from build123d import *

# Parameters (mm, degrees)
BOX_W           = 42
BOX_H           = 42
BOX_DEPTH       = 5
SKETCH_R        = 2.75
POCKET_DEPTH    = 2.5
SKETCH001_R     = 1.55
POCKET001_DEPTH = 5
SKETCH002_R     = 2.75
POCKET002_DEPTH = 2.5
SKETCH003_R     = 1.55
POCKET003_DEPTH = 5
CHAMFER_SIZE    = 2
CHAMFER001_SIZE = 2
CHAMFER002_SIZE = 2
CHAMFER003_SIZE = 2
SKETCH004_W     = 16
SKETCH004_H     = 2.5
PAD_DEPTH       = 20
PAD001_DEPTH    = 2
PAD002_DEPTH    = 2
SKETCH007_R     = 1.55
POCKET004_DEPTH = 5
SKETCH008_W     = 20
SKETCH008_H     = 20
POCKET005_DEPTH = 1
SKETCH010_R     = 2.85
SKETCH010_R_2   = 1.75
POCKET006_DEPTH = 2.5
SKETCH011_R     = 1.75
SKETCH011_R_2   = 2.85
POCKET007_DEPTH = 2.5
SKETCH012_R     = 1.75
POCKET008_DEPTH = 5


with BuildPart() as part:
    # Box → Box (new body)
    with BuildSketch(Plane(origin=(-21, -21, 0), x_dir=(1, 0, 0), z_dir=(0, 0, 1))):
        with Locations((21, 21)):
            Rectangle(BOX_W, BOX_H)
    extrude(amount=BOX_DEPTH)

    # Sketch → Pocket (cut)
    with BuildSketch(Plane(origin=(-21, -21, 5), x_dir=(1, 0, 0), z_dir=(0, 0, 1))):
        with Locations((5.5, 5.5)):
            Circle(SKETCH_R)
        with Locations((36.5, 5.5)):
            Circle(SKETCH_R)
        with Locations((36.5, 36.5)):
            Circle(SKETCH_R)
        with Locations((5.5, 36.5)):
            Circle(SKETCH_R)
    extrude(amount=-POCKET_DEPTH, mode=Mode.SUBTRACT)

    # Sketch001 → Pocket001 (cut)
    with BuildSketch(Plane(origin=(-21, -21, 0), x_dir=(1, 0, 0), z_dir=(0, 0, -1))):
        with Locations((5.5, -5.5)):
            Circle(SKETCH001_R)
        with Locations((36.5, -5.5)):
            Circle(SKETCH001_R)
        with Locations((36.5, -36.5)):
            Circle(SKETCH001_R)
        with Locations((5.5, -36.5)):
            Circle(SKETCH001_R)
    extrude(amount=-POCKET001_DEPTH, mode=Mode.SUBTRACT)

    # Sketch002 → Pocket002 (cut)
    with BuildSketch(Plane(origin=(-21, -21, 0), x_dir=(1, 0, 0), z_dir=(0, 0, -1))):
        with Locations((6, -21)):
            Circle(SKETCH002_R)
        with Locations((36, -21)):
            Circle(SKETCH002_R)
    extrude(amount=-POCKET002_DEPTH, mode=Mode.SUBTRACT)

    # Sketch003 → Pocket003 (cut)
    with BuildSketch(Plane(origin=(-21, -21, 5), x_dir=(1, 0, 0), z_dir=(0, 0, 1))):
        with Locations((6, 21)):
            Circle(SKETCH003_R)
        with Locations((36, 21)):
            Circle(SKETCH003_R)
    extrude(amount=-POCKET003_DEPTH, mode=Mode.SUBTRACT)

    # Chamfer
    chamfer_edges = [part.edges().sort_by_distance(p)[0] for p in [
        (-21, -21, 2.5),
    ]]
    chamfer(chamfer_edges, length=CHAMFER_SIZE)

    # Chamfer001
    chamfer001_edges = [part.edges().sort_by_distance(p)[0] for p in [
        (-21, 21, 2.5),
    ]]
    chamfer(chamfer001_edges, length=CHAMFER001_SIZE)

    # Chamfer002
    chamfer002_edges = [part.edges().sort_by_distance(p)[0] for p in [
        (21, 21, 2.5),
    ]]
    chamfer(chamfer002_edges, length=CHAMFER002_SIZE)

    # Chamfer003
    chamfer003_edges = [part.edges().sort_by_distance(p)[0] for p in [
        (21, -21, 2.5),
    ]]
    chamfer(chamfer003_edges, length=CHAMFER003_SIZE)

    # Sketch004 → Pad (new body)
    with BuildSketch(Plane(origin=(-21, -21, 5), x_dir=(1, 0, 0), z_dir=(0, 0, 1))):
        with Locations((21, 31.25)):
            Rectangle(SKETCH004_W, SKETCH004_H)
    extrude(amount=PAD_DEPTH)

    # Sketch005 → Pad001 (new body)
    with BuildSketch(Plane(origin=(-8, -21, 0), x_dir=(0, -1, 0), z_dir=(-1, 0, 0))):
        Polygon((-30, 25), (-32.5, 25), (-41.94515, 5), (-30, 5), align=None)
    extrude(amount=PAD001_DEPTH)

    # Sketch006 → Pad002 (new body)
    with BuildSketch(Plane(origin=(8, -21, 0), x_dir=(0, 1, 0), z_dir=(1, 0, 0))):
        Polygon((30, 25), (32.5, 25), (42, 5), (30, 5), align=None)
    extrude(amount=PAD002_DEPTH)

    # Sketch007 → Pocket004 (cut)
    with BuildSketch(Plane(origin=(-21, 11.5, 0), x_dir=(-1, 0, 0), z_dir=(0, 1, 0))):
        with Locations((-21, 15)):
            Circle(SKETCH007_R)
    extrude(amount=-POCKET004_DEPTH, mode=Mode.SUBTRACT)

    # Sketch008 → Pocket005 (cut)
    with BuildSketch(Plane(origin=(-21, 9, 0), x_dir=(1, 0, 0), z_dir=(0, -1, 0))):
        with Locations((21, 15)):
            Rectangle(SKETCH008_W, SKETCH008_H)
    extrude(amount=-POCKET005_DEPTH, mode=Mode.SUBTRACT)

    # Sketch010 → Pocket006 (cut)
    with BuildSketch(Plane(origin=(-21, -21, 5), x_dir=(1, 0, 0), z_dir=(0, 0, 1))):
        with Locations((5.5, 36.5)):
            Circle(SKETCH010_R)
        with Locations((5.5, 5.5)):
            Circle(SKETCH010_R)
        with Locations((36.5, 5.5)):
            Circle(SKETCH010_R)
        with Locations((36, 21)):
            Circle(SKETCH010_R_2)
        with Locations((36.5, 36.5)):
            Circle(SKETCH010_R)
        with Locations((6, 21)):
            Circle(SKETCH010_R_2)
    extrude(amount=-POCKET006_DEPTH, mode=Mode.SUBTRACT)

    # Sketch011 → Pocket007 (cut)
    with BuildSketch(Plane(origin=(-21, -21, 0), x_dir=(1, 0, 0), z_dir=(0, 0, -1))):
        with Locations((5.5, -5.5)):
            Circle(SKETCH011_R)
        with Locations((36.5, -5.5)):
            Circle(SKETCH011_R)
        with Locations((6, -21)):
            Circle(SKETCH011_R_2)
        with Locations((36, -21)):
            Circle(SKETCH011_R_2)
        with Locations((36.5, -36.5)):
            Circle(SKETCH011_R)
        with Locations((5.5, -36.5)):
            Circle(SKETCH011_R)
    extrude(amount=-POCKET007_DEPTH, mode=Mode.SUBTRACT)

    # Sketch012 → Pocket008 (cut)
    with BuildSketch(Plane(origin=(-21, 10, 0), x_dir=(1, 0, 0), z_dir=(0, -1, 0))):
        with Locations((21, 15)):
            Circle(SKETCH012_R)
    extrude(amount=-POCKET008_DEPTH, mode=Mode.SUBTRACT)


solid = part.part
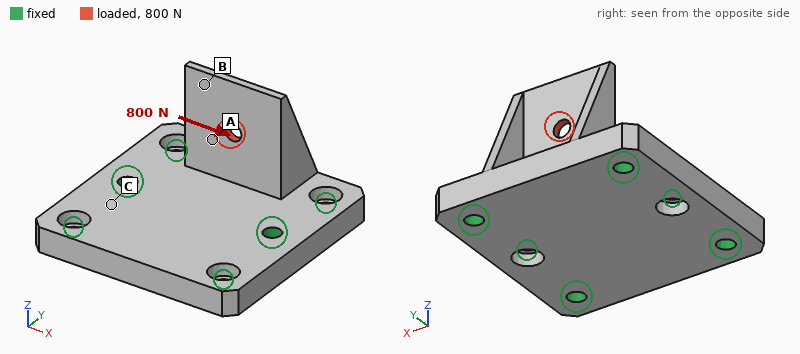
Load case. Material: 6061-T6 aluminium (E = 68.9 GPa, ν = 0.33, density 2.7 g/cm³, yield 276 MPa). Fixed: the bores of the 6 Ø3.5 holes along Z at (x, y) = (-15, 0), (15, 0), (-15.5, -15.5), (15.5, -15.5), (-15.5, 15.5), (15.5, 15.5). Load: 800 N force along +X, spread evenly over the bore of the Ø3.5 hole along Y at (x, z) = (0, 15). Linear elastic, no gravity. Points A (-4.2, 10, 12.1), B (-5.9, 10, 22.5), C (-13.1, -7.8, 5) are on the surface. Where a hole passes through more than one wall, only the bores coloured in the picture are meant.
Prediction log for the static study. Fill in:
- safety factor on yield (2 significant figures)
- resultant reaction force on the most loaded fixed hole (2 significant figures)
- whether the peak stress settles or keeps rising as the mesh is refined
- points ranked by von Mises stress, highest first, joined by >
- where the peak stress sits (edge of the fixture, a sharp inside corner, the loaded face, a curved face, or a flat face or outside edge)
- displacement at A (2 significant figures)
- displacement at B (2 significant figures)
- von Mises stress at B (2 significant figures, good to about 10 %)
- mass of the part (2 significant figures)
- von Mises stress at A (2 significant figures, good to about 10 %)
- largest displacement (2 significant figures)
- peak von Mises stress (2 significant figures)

2.5
420 N
settles
A > B > C
the loaded face
13 µm
26 µm
13 MPa
25 g
45 MPa
32 µm
110 MPa
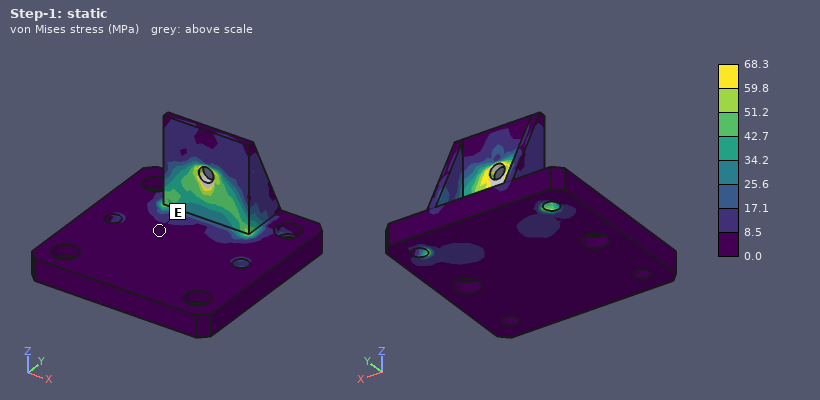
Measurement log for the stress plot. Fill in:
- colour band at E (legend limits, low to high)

0.0 to 8.5 MPa
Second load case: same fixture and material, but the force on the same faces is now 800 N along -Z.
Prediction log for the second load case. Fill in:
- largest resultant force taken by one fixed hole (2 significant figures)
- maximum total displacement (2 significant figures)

340 N
19 µm
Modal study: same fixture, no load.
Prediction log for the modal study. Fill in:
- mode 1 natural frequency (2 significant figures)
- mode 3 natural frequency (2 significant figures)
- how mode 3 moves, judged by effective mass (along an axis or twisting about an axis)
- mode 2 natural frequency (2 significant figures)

11 kHz
19 kHz
along Z
16 kHz
